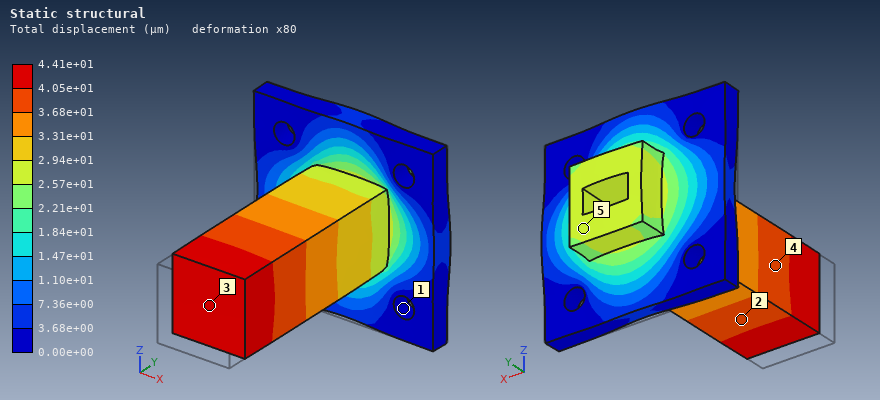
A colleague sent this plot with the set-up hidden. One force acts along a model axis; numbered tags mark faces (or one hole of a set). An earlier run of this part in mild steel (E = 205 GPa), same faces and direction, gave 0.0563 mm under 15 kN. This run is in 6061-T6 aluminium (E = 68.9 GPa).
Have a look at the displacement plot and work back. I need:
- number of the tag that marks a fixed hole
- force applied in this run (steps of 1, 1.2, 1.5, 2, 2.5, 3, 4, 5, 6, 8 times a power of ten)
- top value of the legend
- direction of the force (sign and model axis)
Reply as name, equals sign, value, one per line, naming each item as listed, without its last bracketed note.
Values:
number of the tag that marks a fixed hole = 1
force applied in this run = 4 kN
top value of the legend = 4.41e+01 µm
direction of the force = +Y
